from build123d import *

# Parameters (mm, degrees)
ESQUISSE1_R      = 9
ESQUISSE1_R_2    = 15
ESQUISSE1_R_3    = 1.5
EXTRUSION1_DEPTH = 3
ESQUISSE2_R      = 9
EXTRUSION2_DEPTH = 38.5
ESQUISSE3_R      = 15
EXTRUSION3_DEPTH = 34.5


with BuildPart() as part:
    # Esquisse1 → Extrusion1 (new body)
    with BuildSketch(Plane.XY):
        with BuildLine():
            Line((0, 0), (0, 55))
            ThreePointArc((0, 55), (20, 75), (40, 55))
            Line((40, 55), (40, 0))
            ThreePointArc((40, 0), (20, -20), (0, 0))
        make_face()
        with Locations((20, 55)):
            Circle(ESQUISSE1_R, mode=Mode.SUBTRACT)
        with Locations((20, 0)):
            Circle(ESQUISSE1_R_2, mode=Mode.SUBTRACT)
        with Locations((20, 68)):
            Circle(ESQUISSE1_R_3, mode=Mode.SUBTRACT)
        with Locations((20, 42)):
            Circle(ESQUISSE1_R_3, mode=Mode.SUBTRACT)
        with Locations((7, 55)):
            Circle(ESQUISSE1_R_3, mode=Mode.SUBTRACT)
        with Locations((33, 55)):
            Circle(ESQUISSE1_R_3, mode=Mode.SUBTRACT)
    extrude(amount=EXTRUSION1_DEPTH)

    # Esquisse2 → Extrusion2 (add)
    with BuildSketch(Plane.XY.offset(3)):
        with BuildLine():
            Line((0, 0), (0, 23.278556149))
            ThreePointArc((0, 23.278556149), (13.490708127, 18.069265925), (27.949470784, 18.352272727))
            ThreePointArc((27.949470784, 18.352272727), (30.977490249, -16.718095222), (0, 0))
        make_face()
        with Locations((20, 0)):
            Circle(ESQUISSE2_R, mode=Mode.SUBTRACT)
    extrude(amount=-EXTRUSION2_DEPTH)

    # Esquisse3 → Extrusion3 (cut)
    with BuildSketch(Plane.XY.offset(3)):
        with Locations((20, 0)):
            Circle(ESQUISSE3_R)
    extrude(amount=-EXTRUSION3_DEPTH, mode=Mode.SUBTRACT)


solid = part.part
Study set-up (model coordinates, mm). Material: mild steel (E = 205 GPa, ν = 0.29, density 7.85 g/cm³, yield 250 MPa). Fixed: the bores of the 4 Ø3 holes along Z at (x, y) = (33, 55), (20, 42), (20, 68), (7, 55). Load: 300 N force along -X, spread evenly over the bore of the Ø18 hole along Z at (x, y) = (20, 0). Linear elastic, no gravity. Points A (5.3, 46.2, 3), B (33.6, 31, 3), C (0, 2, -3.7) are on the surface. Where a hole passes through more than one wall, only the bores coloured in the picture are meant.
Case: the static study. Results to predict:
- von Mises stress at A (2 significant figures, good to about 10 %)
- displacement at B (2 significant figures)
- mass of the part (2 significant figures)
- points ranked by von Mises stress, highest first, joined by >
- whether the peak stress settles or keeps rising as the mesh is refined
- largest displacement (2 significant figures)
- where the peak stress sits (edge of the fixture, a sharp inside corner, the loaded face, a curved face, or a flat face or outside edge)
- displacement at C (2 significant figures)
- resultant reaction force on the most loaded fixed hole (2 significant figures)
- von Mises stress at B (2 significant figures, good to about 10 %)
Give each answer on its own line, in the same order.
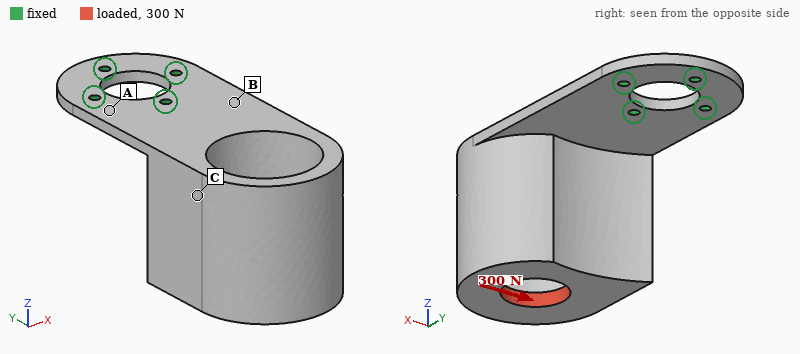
110 MPa
0.059 mm
240 g
A > B > C
keeps rising
0.32 mm
edge of the fixture
0.16 mm
420 N
73 MPa
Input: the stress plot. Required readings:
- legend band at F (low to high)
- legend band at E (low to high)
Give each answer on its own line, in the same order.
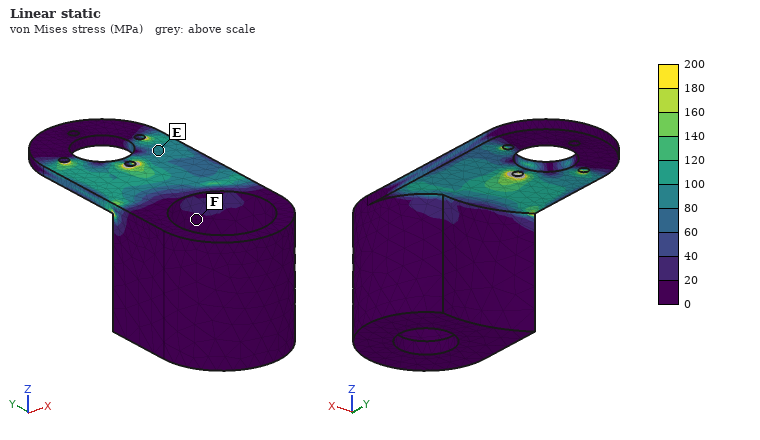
0 to 20 MPa
80 to 100 MPa
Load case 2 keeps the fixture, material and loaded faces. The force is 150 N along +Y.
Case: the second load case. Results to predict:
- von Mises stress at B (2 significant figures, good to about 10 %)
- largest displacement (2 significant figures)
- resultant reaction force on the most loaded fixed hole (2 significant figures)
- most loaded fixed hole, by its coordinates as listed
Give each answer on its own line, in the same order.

76 MPa
0.46 mm
240 N
(20, 42)
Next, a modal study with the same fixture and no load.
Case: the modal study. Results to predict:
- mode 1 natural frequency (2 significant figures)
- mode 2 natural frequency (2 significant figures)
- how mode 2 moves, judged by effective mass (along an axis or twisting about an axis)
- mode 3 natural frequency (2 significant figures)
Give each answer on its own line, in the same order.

240 Hz
520 Hz
along X
1600 Hz
